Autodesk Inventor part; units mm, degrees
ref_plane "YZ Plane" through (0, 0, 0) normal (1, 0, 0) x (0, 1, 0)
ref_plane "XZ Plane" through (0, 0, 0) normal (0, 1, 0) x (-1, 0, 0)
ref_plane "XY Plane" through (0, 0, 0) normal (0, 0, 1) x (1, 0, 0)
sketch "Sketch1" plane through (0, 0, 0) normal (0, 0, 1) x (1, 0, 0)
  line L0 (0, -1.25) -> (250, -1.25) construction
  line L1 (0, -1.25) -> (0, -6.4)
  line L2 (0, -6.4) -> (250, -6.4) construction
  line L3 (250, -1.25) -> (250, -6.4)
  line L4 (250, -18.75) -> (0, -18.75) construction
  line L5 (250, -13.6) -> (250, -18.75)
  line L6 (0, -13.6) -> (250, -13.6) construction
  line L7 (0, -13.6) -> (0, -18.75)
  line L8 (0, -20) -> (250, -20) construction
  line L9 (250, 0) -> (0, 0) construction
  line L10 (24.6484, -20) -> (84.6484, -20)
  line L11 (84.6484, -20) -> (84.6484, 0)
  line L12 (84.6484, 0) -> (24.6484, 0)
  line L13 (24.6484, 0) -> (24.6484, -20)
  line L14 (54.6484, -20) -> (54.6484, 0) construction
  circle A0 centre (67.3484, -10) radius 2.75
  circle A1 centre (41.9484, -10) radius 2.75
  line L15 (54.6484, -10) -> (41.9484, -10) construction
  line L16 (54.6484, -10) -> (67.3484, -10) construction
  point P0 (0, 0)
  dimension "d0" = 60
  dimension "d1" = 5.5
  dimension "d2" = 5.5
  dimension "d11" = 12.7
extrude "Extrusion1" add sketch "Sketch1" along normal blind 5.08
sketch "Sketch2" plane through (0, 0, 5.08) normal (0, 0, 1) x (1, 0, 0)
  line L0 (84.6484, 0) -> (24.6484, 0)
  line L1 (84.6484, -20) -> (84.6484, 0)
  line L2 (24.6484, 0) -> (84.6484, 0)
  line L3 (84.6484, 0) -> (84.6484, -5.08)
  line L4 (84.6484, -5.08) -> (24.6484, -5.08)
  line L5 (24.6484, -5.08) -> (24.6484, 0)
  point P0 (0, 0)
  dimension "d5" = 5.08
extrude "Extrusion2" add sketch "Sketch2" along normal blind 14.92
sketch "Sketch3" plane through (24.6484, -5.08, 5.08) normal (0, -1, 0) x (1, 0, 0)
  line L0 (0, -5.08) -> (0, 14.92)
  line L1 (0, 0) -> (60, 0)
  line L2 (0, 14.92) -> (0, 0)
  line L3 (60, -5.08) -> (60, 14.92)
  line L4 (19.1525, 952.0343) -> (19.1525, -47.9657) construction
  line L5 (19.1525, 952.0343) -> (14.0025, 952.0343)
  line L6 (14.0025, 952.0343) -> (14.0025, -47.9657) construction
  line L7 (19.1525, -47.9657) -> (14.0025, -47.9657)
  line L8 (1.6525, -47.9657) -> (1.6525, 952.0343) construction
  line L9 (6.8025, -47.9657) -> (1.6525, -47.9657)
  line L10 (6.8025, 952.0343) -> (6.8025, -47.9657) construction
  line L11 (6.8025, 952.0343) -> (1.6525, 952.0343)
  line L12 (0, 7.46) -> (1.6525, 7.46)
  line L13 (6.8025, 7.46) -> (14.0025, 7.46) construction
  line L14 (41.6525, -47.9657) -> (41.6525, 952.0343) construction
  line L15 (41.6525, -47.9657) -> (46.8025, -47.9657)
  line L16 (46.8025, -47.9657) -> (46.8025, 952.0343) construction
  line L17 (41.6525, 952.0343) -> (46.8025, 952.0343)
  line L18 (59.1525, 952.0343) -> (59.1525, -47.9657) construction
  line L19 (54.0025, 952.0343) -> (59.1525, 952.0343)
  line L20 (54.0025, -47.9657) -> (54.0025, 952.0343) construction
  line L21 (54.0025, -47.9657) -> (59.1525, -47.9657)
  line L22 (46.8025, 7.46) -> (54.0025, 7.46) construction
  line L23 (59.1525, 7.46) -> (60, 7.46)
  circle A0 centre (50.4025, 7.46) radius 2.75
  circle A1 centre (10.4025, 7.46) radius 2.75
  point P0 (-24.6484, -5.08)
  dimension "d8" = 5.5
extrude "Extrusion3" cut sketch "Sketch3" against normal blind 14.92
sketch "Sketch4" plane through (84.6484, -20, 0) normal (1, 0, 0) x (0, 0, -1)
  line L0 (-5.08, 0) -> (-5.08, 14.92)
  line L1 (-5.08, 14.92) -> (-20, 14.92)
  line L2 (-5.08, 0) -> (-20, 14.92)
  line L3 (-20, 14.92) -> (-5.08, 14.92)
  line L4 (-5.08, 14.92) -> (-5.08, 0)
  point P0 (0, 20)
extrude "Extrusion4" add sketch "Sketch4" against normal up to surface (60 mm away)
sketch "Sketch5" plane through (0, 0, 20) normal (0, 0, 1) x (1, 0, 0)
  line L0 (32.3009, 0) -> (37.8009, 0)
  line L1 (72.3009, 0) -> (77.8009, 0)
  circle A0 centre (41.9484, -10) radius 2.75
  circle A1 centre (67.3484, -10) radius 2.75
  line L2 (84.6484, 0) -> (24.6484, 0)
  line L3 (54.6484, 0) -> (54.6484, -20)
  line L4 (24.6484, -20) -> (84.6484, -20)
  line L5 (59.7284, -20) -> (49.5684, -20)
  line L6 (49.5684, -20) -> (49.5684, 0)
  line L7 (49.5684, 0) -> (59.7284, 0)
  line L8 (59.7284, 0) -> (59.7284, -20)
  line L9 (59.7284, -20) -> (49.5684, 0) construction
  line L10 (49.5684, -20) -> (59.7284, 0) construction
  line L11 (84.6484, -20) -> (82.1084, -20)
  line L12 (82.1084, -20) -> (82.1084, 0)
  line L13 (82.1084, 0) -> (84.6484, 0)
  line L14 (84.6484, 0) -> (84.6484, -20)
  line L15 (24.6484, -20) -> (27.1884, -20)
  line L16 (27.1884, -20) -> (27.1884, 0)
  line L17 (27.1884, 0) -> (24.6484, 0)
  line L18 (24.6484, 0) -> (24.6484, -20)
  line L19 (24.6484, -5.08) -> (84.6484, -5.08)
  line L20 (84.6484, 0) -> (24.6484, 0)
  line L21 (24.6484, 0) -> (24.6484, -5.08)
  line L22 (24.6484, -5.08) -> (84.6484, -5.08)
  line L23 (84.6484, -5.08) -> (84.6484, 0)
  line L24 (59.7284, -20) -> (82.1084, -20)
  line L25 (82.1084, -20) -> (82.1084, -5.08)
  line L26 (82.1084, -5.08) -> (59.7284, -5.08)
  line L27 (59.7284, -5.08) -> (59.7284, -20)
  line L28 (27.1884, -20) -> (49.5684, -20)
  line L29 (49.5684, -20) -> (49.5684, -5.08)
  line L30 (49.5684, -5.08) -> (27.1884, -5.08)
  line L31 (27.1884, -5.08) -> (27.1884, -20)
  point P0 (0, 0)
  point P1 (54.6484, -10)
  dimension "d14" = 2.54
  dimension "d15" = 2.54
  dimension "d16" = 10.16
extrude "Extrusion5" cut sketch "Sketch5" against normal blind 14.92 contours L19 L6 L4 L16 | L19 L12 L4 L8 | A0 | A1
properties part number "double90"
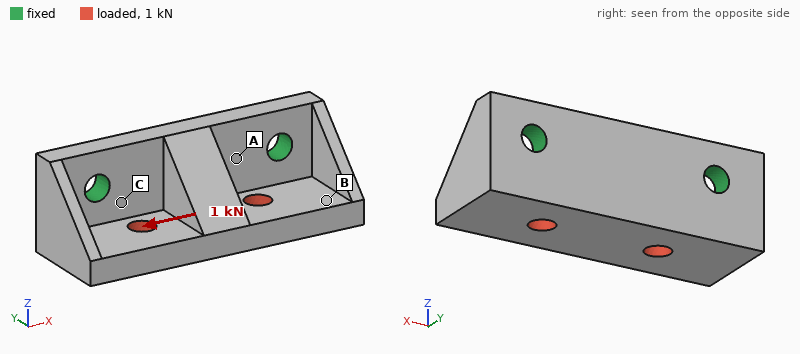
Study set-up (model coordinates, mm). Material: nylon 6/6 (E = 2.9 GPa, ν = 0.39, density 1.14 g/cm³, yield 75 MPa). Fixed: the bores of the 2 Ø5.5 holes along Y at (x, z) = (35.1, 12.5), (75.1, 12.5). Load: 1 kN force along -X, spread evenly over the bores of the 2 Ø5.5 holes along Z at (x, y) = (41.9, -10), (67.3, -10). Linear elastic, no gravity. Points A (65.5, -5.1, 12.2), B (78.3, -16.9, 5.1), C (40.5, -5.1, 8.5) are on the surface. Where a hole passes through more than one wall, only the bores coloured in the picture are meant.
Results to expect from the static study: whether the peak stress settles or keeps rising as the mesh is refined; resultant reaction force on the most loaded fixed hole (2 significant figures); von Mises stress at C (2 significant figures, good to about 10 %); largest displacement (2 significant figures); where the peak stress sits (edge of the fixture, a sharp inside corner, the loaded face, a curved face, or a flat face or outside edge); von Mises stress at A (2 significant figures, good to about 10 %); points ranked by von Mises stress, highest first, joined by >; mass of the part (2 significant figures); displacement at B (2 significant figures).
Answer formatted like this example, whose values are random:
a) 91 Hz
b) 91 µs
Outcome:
a) keeps rising
b) 570 N
c) 11 MPa
d) 0.14 mm
e) edge of the fixture
f) 7.0 MPa
g) C > A > B
h) 14 g
i) 0.11 mm
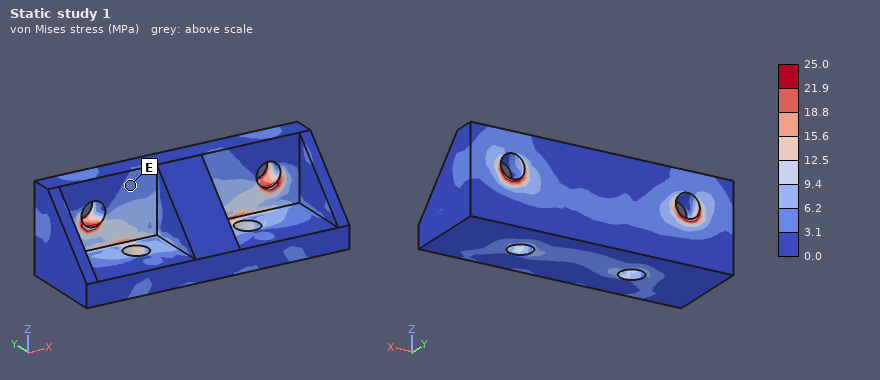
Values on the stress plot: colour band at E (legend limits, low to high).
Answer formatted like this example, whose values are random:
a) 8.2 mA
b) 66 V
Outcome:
a) 3.1 to 6.2 MPa
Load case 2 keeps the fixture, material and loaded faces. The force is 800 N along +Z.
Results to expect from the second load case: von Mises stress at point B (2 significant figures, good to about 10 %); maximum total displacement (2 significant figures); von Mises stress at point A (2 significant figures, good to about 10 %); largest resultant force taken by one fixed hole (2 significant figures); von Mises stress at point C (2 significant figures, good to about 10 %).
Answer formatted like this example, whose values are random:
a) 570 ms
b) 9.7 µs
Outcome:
a) 4.2 MPa
b) 0.50 mm
c) 14 MPa
d) 430 N
e) 22 MPa
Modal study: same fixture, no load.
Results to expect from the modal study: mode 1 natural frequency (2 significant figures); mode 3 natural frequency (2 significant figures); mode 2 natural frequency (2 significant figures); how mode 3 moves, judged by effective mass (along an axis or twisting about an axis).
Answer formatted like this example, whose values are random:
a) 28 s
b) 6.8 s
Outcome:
a) 2500 Hz
b) 4700 Hz
c) 3800 Hz
d) along Y
